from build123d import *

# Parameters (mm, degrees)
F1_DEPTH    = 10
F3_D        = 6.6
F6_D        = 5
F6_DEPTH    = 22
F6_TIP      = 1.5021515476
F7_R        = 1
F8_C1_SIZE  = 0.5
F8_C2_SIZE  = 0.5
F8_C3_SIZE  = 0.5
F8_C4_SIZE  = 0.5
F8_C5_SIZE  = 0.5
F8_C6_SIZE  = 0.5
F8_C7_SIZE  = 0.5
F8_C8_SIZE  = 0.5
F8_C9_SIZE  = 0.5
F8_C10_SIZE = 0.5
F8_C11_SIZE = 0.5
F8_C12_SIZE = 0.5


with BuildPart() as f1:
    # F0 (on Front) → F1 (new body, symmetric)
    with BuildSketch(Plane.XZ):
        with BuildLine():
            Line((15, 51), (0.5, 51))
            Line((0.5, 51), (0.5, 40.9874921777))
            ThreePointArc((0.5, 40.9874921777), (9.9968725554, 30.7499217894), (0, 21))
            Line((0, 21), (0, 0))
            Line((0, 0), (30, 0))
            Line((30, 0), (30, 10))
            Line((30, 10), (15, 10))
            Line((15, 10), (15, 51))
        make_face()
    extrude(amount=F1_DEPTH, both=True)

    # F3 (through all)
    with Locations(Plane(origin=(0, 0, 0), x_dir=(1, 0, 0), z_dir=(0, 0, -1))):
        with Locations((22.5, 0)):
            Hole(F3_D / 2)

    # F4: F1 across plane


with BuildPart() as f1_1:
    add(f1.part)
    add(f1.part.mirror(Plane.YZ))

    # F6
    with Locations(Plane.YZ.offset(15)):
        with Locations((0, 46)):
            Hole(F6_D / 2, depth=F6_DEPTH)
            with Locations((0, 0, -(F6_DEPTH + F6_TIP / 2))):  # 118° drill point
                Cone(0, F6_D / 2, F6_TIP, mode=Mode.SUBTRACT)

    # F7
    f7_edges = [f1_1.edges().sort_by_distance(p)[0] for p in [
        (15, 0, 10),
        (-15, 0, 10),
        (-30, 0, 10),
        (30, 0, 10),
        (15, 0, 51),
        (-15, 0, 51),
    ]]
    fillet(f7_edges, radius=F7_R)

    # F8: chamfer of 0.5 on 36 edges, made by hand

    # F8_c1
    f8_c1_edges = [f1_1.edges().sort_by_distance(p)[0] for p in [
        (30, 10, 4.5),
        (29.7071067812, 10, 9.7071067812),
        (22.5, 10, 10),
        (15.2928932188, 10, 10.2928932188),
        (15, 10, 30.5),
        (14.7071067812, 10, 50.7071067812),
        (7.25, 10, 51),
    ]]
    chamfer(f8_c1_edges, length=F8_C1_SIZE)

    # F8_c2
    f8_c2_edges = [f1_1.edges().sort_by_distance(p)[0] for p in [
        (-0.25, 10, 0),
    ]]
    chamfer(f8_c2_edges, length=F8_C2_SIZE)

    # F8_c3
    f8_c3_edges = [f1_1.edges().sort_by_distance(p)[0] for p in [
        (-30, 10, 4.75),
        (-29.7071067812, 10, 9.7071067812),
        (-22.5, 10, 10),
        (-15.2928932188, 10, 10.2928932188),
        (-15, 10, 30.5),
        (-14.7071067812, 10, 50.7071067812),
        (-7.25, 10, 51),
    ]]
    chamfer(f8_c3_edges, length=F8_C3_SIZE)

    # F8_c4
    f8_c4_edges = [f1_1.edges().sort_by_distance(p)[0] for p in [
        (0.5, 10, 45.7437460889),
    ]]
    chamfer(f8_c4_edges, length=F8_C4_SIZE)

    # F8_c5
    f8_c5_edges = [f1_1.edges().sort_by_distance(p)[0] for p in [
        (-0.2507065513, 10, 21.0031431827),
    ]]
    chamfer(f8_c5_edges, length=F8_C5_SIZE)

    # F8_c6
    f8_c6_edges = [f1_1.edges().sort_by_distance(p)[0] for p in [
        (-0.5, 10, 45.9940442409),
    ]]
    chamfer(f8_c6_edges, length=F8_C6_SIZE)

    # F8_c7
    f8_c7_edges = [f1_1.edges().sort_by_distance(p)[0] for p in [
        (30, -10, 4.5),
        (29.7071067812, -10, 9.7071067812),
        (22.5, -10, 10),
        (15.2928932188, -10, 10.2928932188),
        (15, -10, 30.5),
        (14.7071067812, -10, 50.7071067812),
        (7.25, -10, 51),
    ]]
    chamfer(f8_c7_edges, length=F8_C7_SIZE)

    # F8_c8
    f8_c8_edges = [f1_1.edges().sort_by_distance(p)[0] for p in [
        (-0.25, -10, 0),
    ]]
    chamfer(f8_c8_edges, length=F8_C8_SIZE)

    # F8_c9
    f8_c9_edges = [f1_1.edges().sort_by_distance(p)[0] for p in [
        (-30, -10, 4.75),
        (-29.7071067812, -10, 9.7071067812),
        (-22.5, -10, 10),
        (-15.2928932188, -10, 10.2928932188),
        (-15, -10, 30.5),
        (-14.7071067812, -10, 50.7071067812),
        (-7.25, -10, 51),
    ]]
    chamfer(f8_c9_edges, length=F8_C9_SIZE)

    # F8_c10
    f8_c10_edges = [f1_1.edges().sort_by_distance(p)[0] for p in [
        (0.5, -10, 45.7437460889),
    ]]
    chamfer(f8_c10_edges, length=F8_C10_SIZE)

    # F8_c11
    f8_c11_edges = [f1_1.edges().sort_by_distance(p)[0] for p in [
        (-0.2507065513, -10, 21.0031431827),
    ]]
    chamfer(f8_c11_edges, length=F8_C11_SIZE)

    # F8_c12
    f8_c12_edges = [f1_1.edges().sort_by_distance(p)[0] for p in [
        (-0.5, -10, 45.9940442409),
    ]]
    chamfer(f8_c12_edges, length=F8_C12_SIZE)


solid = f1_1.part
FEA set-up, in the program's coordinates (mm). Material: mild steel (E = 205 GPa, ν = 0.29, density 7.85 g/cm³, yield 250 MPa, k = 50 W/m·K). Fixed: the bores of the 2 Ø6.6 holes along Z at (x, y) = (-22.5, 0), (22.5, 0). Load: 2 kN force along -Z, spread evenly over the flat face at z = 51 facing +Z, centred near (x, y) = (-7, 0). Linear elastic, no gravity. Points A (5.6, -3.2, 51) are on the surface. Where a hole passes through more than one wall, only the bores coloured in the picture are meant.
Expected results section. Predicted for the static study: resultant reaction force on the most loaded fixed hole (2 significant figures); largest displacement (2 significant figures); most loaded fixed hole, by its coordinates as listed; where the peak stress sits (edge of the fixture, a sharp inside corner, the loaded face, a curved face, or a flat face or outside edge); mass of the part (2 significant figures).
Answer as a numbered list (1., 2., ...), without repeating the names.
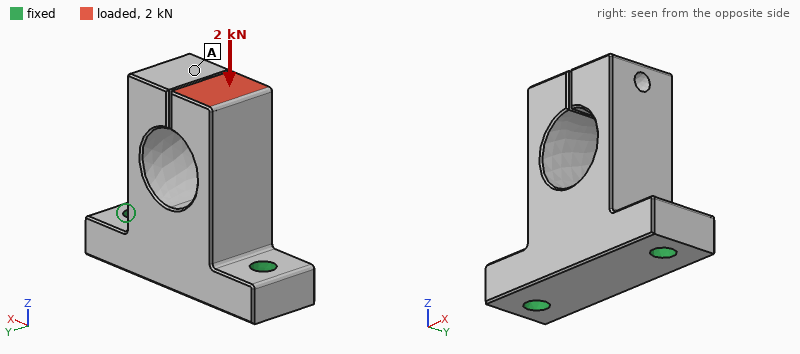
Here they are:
1. 1.5 kN
2. 65 µm
3. (-22.5, 0)
4. a curved face
5. 230 g
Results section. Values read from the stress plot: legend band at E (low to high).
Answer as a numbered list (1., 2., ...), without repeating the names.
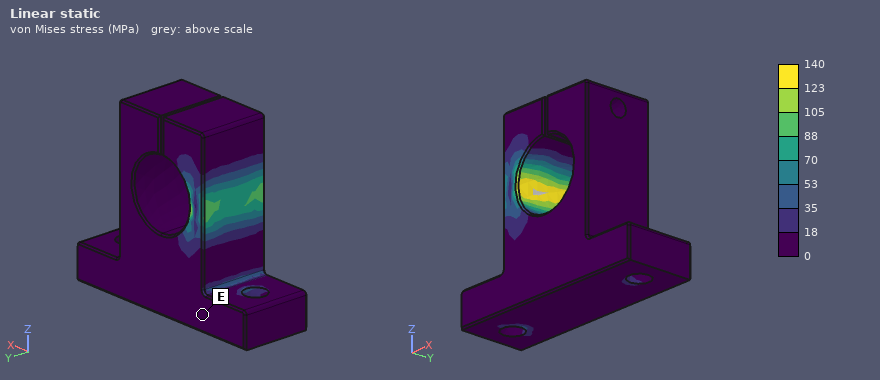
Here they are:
1. 0 to 18 MPa
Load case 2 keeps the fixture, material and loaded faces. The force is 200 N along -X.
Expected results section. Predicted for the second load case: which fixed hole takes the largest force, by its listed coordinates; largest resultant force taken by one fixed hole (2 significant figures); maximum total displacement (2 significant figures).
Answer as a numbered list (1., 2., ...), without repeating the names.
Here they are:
1. (22.5, 0)
2. 310 N
3. 31 µm
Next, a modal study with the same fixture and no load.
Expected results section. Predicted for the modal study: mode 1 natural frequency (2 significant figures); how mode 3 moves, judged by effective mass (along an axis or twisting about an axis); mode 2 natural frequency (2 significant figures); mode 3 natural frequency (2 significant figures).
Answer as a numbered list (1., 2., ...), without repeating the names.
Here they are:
1. 3300 Hz
2. along Y
3. 3400 Hz
4. 3600 Hz
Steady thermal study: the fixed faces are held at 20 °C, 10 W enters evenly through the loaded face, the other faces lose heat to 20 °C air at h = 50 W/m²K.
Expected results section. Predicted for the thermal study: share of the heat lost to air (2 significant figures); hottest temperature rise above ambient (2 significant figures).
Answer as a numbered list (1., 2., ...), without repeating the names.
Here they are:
1. 38 %
2. 44 K
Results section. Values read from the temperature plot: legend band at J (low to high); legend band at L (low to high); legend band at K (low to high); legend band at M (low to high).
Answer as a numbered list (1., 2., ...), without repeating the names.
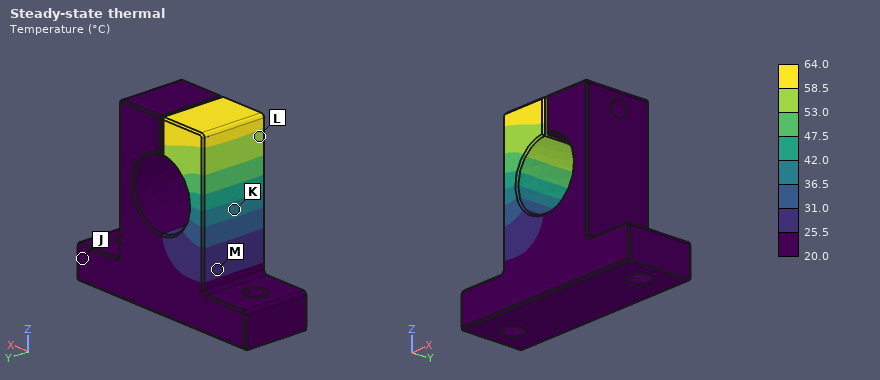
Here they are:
1. 20.0 to 25.5 °C
2. 53.0 to 58.5 °C
3. 36.5 to 42.0 °C
4. 25.5 to 31.0 °C
